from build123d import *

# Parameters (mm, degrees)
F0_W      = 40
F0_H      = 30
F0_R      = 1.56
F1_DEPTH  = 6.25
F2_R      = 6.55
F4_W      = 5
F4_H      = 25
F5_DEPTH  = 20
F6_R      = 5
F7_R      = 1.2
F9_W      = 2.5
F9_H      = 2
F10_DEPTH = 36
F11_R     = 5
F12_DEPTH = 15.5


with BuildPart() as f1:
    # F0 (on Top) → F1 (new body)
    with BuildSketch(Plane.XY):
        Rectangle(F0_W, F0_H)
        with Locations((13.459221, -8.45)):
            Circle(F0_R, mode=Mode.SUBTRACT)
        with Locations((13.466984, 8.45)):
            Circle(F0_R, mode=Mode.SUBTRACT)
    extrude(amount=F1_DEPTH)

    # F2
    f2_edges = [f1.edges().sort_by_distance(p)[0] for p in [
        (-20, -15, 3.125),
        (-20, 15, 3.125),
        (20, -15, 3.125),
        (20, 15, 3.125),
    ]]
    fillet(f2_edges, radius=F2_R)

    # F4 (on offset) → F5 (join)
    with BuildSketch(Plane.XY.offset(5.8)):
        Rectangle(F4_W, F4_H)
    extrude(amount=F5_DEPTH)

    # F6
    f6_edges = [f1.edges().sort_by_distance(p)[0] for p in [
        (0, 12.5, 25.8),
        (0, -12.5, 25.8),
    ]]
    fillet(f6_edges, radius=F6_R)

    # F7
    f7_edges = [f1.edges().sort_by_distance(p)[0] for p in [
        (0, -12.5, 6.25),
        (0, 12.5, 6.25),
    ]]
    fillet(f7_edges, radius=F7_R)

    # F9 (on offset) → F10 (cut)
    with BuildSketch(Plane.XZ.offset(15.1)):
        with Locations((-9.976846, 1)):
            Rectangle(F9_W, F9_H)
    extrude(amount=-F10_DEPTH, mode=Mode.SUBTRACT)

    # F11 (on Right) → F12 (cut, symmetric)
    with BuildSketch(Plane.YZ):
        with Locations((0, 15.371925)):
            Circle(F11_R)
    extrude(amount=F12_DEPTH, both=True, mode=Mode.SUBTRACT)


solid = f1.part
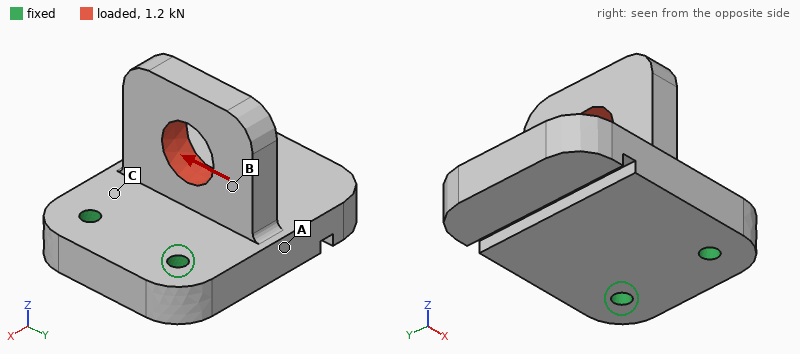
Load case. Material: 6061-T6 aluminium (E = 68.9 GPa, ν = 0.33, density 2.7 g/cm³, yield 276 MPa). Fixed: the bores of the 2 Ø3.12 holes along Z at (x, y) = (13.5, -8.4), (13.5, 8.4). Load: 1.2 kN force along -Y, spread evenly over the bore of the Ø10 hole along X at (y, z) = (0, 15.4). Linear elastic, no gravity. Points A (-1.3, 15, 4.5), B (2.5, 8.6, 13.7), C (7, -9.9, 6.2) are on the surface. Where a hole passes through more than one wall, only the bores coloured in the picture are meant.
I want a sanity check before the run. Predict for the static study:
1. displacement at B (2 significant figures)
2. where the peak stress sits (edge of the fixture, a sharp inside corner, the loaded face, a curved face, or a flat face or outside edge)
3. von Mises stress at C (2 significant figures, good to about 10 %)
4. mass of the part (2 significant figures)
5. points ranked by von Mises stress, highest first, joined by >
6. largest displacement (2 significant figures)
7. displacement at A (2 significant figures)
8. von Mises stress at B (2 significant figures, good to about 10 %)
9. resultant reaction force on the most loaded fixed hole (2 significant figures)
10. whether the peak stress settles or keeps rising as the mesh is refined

30 µm
edge of the fixture
39 MPa
24 g
C > B > A
54 µm
25 µm
29 MPa
1.2 kN
keeps rising
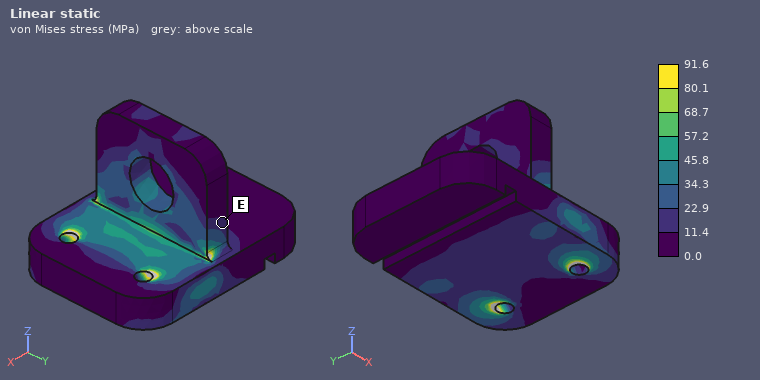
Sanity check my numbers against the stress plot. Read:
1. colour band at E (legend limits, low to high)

11.4 to 22.9 MPa
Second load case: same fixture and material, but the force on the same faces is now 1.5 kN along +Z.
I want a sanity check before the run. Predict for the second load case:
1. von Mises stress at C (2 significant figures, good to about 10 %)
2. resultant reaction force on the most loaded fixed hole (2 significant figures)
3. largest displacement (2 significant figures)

55 MPa
750 N
0.11 mm
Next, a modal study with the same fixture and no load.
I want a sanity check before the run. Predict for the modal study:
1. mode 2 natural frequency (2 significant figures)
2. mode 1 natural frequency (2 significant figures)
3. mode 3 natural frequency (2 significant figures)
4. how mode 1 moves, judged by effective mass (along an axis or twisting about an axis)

8700 Hz
3800 Hz
9300 Hz
along Z
